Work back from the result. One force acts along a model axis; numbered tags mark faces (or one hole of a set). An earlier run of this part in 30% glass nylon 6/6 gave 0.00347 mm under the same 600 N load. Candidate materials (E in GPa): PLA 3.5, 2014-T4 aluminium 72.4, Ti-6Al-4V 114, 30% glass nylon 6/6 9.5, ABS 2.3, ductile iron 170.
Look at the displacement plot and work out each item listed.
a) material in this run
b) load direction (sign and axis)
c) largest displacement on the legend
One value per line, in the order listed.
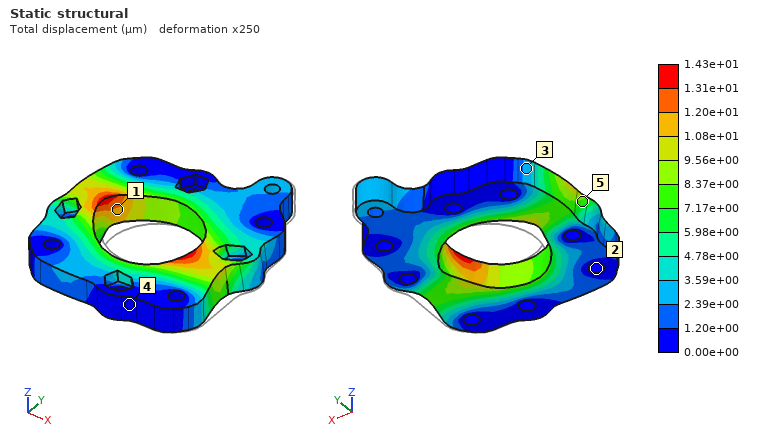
ABS
-X
1.43e+01 µm
